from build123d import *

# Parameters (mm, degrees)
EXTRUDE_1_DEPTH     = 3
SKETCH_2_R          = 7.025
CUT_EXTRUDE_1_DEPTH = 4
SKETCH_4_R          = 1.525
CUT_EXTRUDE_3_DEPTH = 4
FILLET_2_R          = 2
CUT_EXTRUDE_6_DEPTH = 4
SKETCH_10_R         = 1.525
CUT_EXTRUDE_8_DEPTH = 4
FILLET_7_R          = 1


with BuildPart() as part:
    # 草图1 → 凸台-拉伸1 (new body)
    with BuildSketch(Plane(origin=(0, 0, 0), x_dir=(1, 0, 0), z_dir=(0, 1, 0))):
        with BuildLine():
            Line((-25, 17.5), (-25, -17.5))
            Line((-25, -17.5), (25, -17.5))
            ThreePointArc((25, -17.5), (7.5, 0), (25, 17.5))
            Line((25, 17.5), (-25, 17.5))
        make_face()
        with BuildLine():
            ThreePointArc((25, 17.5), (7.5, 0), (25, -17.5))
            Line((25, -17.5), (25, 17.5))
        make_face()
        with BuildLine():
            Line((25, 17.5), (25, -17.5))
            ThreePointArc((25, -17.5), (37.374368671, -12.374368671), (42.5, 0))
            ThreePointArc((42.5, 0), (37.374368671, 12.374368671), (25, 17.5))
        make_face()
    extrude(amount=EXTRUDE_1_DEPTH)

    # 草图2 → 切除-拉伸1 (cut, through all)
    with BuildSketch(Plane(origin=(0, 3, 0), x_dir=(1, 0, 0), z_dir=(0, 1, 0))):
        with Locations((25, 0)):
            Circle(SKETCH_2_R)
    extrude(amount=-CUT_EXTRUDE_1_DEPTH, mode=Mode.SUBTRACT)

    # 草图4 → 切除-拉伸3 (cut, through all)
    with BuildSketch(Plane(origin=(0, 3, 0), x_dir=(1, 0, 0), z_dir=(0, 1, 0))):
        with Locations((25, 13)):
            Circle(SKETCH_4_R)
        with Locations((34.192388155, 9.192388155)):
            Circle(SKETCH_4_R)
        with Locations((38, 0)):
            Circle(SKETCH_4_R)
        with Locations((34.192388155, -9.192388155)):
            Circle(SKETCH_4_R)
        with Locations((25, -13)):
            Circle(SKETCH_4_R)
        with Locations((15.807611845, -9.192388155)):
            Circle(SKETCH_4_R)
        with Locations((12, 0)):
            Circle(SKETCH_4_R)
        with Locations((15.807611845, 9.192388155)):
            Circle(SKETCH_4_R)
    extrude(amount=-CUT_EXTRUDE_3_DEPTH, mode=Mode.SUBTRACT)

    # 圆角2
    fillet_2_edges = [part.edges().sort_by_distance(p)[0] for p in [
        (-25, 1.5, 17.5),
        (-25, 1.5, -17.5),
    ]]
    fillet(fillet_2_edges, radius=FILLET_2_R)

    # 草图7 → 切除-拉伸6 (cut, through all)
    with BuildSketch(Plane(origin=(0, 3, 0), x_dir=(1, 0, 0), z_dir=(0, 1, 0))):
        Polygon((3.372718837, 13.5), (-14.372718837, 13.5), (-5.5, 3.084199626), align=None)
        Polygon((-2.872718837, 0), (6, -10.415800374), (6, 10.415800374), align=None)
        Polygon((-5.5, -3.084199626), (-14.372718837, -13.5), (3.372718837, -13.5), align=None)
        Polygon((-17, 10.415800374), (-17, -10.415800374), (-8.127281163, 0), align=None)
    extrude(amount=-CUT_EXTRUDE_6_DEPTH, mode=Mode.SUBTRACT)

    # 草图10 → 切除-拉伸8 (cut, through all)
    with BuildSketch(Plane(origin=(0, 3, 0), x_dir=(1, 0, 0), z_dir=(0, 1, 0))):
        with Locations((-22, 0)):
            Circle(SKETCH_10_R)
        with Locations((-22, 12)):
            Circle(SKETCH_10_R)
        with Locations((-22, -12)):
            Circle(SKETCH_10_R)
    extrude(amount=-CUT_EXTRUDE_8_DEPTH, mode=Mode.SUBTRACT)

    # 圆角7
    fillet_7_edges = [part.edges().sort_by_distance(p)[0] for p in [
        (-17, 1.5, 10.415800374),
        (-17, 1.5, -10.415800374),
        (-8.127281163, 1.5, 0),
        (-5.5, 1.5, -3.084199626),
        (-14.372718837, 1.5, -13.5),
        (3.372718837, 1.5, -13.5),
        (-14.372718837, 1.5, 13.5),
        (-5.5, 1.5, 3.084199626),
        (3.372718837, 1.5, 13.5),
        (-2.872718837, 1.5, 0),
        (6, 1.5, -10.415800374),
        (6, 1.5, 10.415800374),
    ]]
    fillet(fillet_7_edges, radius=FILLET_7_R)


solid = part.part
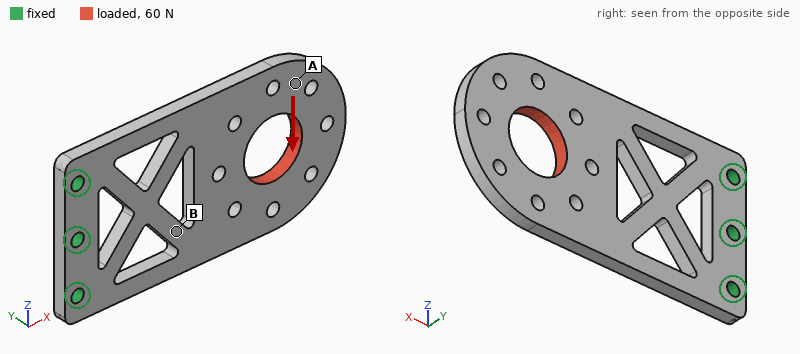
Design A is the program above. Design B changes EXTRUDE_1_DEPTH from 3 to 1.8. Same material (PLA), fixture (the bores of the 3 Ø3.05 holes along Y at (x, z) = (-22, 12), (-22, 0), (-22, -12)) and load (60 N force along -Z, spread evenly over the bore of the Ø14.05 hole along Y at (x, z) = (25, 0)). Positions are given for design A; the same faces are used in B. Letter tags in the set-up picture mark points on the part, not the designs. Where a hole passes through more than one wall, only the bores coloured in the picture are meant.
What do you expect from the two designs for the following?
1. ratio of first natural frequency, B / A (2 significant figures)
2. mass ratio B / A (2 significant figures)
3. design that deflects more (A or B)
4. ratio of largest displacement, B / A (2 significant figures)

0.62
0.60
B
1.7
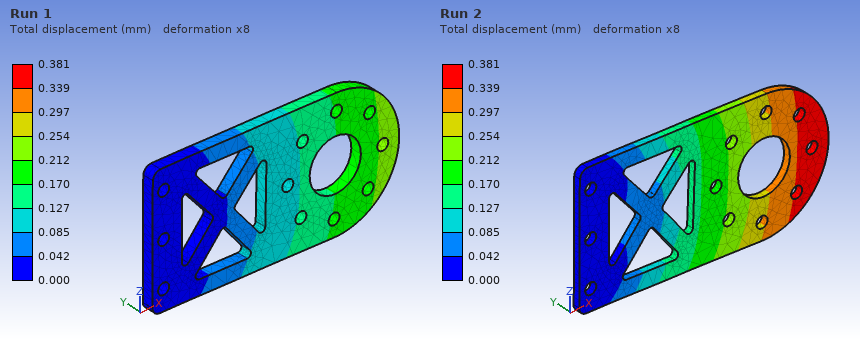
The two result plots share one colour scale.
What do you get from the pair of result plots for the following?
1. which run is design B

Run 2
